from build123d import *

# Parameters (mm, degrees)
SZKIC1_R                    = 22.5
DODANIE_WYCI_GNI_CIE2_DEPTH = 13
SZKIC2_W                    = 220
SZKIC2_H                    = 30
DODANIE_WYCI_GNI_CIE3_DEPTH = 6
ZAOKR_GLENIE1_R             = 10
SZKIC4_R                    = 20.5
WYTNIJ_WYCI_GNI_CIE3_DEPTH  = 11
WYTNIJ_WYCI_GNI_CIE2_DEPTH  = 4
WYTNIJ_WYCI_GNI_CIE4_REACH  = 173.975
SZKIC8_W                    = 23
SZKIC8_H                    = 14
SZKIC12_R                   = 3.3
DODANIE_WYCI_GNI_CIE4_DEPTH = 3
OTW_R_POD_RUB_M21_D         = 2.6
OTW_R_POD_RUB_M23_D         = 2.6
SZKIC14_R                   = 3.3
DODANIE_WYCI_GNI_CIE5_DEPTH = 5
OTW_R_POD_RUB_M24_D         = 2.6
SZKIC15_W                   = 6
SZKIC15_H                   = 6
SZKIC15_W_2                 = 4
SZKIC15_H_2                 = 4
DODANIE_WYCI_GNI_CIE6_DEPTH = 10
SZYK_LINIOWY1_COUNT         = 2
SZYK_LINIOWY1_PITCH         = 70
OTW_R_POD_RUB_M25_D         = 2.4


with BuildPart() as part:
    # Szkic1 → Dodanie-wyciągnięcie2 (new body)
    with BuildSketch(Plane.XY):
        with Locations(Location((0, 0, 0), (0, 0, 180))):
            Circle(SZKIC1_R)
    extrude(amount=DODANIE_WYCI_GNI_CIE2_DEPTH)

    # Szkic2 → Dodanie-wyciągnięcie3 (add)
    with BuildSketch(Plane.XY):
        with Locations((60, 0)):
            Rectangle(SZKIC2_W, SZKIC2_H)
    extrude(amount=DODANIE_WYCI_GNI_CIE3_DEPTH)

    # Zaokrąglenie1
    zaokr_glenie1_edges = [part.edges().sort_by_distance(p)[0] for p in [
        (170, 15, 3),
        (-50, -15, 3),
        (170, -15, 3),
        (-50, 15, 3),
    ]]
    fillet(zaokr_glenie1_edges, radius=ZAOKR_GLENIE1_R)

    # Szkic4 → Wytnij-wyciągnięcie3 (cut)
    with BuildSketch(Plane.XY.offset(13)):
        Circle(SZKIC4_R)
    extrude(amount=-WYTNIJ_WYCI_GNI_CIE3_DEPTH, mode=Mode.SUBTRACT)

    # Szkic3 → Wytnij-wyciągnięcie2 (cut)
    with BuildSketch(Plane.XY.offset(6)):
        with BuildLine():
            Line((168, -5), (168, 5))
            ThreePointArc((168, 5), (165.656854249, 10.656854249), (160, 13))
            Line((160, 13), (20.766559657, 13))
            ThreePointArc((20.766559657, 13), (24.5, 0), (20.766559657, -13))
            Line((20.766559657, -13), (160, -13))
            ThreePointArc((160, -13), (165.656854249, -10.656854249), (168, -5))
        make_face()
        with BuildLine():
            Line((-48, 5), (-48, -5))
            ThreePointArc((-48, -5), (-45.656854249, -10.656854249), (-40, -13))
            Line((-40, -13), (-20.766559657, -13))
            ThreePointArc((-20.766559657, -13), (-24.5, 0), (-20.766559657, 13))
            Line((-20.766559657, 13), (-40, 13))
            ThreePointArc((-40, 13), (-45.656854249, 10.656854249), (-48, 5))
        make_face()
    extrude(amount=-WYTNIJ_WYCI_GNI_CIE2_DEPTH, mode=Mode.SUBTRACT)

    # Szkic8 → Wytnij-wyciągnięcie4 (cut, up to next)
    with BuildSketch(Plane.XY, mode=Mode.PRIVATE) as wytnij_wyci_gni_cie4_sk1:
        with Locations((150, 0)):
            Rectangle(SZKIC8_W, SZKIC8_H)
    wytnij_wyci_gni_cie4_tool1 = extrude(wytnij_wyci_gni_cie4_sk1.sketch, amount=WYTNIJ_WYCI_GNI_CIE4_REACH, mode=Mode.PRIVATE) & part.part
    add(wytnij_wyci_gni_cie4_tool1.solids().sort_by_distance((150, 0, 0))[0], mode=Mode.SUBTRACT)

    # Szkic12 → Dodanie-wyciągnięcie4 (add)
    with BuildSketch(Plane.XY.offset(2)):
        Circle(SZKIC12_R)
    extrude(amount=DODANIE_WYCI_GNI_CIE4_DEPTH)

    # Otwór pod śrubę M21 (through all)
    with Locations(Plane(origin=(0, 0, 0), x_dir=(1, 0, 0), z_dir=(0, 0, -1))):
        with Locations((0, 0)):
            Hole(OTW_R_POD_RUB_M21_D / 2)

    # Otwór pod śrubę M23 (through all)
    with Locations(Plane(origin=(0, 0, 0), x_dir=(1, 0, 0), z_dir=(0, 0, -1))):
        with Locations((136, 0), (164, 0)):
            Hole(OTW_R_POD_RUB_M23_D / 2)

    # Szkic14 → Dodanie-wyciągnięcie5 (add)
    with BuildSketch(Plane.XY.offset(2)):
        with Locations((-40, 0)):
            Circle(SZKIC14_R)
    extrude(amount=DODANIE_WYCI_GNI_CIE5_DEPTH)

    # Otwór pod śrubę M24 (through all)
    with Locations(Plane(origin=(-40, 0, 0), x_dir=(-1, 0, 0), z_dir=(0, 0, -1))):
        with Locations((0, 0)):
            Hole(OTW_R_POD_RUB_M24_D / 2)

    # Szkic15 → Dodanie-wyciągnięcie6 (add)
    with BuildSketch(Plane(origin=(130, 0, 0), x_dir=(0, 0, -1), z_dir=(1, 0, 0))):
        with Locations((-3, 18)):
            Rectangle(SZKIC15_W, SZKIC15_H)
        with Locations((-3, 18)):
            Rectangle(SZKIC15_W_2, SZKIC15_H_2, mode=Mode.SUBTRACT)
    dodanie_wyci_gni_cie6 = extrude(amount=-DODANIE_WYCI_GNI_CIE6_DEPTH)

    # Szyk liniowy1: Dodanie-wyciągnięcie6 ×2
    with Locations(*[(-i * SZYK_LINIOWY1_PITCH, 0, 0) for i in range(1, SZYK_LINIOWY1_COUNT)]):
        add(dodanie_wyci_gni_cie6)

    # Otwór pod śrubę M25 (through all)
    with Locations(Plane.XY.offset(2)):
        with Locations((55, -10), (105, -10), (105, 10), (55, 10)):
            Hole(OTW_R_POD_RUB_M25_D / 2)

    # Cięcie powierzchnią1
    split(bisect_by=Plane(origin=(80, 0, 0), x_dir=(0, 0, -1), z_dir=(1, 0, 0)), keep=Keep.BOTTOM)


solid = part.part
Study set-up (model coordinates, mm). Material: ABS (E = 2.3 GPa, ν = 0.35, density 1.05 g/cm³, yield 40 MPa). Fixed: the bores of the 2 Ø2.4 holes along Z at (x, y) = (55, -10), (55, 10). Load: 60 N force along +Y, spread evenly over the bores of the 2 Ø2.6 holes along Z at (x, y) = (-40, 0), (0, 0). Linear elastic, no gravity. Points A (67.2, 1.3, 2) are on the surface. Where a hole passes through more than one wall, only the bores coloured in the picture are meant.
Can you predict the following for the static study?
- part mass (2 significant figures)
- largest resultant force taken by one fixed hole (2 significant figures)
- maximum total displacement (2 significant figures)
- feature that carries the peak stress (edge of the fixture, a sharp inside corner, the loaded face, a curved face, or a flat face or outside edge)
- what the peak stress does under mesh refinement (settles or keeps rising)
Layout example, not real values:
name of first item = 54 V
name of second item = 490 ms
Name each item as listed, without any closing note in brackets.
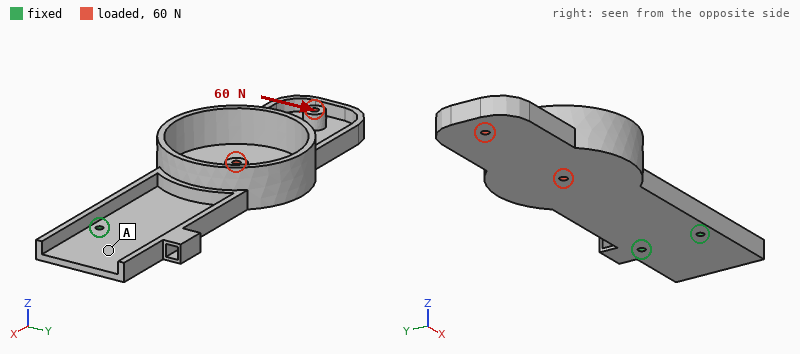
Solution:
part mass = 15 g
largest resultant force taken by one fixed hole = 230 N
maximum total displacement = 1.4 mm
feature that carries the peak stress = edge of the fixture
what the peak stress does under mesh refinement = keeps rising
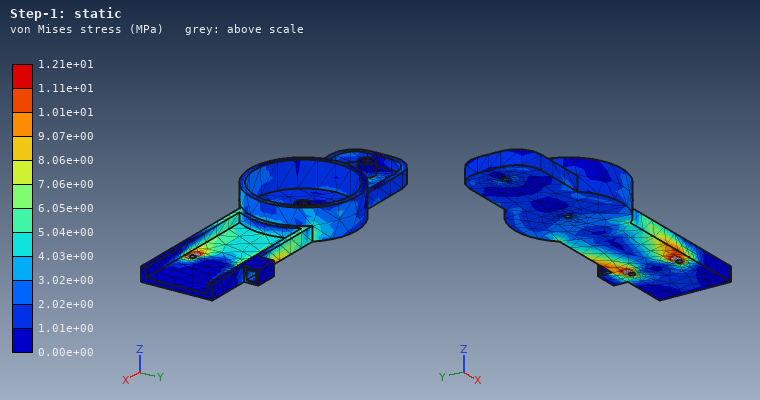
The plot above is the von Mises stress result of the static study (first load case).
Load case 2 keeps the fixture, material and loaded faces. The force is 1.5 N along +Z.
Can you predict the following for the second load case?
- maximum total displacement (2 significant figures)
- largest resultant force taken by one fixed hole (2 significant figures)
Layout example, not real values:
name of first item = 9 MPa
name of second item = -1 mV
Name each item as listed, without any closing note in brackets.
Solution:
maximum total displacement = 1.4 mm
largest resultant force taken by one fixed hole = 1.3 N
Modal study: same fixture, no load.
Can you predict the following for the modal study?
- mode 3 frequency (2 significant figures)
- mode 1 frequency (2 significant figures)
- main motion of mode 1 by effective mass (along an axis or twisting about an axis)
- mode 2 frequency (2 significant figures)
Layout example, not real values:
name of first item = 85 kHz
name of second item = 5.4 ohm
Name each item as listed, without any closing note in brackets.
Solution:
mode 3 frequency = 500 Hz
mode 1 frequency = 75 Hz
main motion of mode 1 by effective mass = along Z
mode 2 frequency = 290 Hz
